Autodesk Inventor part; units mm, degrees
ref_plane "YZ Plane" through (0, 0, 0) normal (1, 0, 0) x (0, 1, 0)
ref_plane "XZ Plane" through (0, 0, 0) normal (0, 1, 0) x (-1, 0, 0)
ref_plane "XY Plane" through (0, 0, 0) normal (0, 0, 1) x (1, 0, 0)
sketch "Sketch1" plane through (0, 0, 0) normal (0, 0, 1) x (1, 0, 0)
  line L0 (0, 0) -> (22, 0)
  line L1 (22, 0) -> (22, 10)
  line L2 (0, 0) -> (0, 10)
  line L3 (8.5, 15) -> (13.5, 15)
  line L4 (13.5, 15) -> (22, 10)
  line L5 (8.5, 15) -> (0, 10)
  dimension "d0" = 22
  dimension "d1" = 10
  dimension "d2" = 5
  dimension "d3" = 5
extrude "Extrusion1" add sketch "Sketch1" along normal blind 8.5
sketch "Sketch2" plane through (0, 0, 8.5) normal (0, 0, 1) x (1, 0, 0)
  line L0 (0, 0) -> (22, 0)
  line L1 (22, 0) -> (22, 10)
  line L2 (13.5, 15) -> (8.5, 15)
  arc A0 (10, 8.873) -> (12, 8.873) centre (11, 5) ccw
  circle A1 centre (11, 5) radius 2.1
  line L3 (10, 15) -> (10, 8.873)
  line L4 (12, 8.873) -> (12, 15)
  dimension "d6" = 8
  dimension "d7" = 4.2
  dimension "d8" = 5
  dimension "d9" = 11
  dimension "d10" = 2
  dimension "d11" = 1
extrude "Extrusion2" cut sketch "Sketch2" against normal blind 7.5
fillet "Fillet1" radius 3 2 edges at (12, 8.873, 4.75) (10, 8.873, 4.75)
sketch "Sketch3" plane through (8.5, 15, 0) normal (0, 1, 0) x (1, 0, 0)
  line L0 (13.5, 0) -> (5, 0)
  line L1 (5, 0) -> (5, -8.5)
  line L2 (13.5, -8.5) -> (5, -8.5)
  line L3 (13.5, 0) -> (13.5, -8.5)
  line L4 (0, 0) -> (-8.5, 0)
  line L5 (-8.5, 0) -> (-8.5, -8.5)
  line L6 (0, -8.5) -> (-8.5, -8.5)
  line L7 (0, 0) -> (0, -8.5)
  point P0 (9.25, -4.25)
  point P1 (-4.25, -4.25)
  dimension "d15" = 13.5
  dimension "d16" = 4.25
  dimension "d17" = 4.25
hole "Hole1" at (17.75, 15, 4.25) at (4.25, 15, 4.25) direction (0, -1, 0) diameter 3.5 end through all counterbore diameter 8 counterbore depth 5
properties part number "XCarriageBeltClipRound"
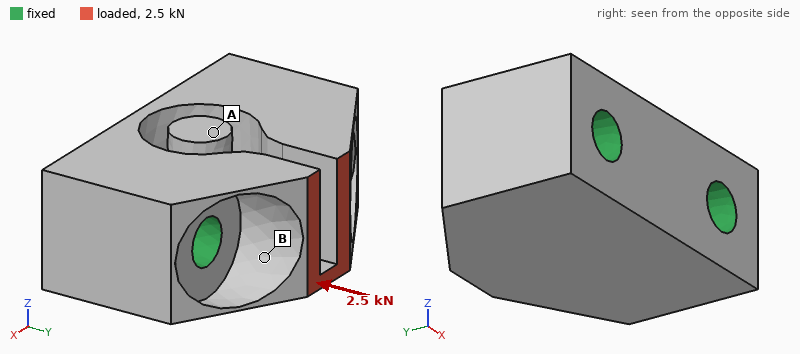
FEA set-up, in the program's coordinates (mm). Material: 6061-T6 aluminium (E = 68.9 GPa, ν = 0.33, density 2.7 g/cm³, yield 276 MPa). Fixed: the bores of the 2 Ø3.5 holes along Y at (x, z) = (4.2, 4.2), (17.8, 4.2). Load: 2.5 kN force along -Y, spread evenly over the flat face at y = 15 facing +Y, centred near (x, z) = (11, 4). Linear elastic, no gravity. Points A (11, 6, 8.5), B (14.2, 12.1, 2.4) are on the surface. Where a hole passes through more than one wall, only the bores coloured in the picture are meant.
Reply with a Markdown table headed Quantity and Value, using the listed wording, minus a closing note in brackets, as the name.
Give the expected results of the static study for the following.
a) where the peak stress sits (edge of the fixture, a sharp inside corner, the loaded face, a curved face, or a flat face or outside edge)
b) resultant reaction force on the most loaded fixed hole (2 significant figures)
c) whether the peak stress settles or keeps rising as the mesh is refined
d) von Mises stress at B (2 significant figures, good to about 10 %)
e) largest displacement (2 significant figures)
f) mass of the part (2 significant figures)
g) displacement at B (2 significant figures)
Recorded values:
| Quantity | Value |
|---|---|
| where the peak stress sits | a sharp inside corner |
| resultant reaction force on the most loaded fixed hole | 1.3 kN |
| whether the peak stress settles or keeps rising as the mesh is refined | keeps rising |
| von Mises stress at B | 64 MPa |
| largest displacement | 36 µm |
| mass of the part | 4.4 g |
| displacement at B | 10.0 µm |
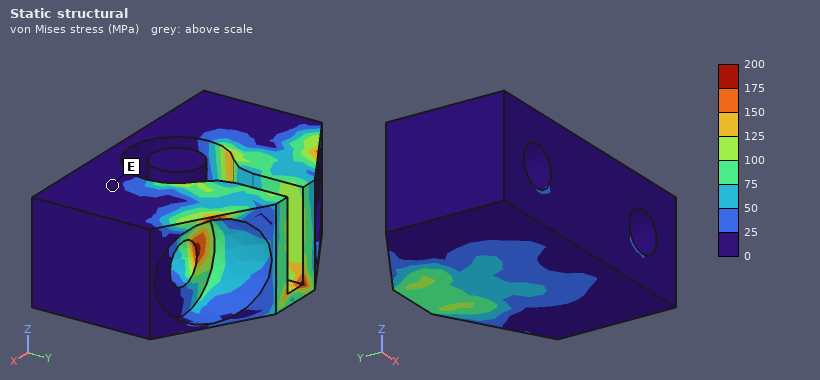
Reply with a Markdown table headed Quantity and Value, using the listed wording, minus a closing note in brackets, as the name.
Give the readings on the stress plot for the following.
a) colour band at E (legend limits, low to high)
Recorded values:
| Quantity | Value |
|---|---|
| colour band at E | 0 to 25 MPa |
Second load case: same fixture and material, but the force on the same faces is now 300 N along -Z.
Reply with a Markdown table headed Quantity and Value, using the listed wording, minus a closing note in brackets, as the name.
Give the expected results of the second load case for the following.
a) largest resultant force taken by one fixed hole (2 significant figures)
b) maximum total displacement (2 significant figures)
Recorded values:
| Quantity | Value |
|---|---|
| largest resultant force taken by one fixed hole | 150 N |
| maximum total displacement | 9.5 µm |
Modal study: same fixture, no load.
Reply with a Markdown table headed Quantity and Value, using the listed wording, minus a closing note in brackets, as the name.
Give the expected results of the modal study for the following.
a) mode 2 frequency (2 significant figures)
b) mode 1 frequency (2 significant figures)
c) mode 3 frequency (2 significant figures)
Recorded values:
| Quantity | Value |
|---|---|
| mode 2 frequency | 26 kHz |
| mode 1 frequency | 25 kHz |
| mode 3 frequency | 51 kHz |
